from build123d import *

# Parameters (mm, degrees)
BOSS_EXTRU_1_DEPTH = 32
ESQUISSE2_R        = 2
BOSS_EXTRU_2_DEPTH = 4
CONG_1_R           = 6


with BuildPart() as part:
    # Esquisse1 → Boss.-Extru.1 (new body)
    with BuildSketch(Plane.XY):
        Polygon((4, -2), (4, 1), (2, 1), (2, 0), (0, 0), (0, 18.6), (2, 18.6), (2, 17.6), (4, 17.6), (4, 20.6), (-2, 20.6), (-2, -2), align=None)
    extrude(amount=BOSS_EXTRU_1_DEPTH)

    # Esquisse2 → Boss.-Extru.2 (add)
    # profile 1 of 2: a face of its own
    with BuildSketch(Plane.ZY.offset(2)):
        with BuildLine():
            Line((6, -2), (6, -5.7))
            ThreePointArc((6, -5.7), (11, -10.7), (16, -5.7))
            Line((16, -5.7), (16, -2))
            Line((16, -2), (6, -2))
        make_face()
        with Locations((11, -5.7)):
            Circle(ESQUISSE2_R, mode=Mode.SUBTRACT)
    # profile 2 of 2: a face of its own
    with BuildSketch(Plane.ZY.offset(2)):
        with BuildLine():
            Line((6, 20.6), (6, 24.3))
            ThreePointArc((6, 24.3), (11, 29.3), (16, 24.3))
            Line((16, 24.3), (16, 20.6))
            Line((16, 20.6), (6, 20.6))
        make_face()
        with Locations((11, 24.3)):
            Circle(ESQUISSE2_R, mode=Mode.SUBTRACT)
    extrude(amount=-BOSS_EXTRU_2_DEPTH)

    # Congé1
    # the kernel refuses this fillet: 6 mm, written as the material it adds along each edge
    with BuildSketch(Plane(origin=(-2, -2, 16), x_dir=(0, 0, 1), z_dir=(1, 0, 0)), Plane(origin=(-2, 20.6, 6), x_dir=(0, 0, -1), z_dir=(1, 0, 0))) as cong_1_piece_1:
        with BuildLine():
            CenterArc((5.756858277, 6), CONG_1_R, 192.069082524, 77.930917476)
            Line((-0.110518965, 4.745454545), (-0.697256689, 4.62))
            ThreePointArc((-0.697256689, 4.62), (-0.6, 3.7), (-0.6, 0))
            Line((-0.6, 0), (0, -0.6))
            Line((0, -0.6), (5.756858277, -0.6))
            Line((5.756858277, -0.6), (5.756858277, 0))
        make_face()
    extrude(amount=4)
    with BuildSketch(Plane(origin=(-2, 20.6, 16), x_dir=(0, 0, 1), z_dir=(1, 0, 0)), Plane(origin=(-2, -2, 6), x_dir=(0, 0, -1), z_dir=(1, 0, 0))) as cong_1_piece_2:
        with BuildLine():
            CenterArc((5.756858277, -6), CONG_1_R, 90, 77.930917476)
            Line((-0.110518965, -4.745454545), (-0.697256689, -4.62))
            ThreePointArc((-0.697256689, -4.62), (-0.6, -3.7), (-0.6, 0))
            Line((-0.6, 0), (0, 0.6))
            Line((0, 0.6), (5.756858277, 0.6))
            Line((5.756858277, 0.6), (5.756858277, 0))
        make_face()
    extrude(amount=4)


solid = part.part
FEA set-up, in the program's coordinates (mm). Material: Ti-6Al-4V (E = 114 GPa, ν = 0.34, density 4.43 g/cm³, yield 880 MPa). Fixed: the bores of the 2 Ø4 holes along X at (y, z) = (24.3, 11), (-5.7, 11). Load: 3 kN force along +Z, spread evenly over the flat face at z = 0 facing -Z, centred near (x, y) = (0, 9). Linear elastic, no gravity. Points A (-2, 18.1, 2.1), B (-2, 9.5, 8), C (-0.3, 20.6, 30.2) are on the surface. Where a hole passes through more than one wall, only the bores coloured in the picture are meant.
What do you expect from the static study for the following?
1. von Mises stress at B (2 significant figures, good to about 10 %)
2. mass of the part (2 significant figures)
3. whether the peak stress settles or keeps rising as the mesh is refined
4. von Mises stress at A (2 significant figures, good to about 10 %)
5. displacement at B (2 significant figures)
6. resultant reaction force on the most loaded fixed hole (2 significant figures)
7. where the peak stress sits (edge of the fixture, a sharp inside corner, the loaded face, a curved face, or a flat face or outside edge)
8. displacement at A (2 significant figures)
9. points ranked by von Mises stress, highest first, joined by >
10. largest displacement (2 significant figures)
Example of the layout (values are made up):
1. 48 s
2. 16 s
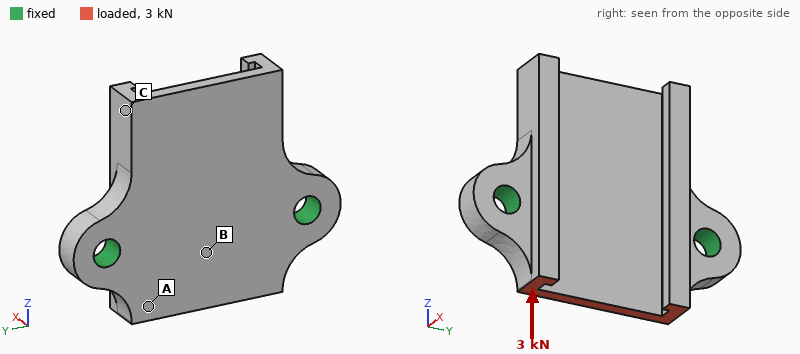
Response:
1. 28 MPa
2. 12 g
3. keeps rising
4. 50 MPa
5. 8.7 µm
6. 1.5 kN
7. edge of the fixture
8. 7.0 µm
9. A > B > C
10. 12 µm
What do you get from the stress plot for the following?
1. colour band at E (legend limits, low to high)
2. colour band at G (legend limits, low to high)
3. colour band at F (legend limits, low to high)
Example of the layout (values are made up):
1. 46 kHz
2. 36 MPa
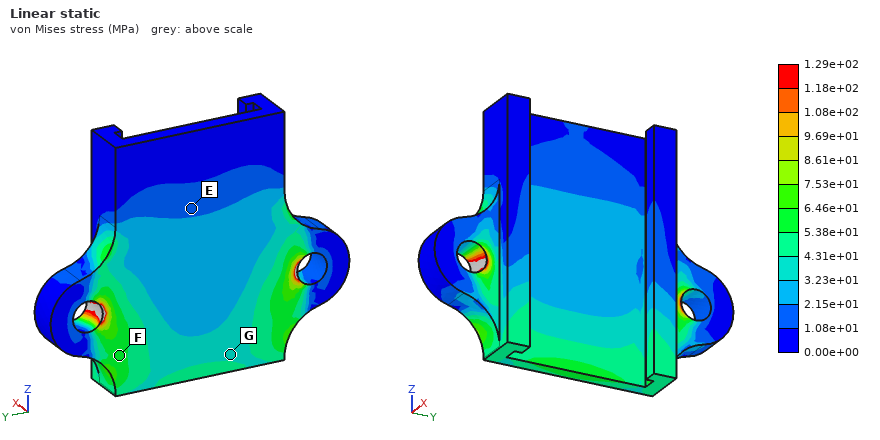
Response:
1. 1.08e+01 to 2.15e+01 MPa
2. 3.23e+01 to 4.31e+01 MPa
3. 5.38e+01 to 6.46e+01 MPa
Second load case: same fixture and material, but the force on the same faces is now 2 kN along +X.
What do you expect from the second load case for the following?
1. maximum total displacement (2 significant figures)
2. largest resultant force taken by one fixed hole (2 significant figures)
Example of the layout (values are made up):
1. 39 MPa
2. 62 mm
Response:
1. 0.21 mm
2. 1.1 kN
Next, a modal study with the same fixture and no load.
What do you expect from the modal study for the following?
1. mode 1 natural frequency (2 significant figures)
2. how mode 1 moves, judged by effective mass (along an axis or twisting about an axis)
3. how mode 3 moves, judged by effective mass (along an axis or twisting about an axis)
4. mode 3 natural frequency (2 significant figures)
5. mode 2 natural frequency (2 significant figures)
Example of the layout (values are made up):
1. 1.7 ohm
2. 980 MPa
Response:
1. 7700 Hz
2. along X
3. along X
4. 17 kHz
5. 13 kHz
